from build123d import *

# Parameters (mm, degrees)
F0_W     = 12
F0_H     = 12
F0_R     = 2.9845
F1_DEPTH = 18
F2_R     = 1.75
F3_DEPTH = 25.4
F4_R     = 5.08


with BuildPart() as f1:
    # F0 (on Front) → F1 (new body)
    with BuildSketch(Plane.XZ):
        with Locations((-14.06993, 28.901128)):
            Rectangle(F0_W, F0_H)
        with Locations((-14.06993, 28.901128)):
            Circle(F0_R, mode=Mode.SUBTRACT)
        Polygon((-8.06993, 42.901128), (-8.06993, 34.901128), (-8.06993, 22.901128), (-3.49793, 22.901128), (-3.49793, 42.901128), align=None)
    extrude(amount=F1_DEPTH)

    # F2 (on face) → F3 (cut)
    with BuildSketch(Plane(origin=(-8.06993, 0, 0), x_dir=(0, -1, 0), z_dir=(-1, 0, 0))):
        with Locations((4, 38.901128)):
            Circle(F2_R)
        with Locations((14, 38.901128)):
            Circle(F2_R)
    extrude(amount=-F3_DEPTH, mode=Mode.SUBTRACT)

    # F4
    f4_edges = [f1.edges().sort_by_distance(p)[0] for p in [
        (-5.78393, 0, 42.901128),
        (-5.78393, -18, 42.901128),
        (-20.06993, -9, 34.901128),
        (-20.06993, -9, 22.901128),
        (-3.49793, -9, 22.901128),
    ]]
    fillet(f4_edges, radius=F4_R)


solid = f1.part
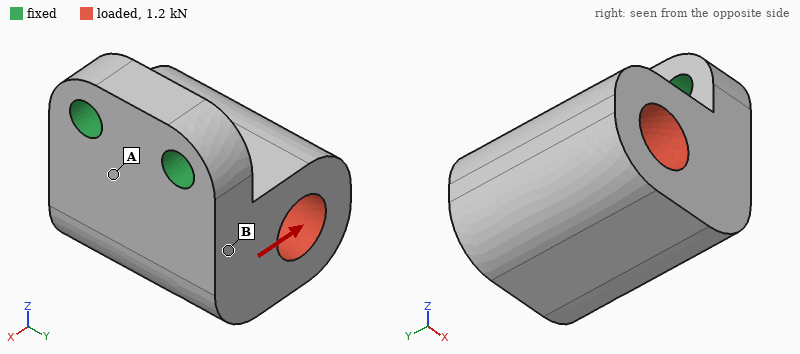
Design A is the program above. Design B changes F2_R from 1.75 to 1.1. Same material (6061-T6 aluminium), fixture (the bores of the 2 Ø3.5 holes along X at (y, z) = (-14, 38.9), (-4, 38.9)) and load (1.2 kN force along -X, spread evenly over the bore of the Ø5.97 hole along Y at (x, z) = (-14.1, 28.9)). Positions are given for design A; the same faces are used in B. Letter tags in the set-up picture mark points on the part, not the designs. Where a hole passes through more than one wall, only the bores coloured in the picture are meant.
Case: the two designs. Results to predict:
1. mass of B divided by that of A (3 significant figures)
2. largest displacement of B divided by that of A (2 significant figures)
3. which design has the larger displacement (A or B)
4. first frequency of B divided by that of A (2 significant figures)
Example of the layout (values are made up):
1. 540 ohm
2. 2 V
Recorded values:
1. 1.02
2. 1.3
3. B
4. 0.89
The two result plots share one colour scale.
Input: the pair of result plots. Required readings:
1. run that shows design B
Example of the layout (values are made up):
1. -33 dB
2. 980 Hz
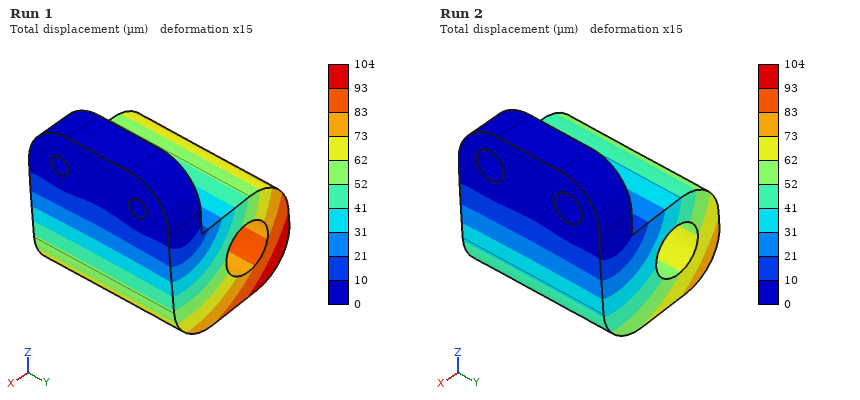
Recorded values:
1. Run 1
